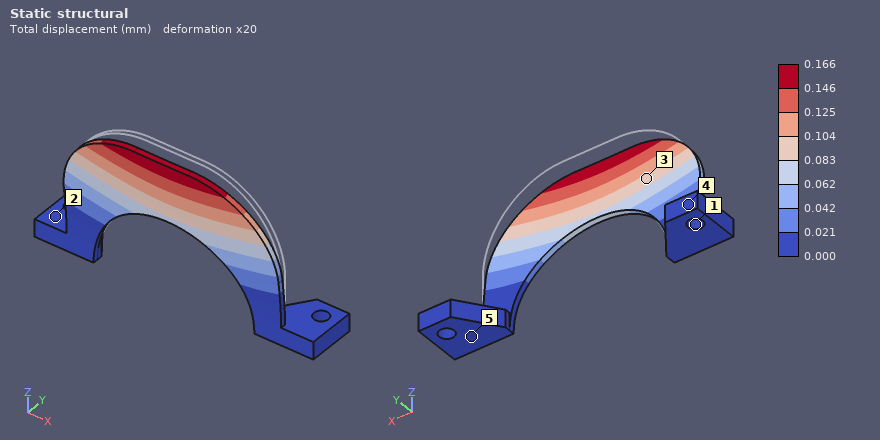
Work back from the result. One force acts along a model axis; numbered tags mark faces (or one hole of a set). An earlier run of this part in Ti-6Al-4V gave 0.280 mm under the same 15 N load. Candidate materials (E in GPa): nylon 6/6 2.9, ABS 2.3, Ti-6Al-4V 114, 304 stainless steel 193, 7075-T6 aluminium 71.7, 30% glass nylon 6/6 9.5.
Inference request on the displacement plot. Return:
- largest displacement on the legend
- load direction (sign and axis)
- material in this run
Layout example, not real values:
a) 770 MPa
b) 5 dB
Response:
a) 0.166 mm
b) -Y
c) 304 stainless steel
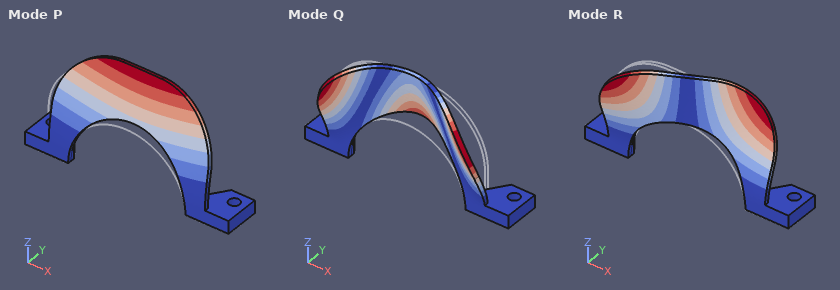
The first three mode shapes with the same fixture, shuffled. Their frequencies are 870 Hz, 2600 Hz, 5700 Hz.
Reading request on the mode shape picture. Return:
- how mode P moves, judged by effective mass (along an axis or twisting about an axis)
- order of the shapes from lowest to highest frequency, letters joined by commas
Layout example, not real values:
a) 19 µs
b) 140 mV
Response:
a) along Y
b) P, R, Q
